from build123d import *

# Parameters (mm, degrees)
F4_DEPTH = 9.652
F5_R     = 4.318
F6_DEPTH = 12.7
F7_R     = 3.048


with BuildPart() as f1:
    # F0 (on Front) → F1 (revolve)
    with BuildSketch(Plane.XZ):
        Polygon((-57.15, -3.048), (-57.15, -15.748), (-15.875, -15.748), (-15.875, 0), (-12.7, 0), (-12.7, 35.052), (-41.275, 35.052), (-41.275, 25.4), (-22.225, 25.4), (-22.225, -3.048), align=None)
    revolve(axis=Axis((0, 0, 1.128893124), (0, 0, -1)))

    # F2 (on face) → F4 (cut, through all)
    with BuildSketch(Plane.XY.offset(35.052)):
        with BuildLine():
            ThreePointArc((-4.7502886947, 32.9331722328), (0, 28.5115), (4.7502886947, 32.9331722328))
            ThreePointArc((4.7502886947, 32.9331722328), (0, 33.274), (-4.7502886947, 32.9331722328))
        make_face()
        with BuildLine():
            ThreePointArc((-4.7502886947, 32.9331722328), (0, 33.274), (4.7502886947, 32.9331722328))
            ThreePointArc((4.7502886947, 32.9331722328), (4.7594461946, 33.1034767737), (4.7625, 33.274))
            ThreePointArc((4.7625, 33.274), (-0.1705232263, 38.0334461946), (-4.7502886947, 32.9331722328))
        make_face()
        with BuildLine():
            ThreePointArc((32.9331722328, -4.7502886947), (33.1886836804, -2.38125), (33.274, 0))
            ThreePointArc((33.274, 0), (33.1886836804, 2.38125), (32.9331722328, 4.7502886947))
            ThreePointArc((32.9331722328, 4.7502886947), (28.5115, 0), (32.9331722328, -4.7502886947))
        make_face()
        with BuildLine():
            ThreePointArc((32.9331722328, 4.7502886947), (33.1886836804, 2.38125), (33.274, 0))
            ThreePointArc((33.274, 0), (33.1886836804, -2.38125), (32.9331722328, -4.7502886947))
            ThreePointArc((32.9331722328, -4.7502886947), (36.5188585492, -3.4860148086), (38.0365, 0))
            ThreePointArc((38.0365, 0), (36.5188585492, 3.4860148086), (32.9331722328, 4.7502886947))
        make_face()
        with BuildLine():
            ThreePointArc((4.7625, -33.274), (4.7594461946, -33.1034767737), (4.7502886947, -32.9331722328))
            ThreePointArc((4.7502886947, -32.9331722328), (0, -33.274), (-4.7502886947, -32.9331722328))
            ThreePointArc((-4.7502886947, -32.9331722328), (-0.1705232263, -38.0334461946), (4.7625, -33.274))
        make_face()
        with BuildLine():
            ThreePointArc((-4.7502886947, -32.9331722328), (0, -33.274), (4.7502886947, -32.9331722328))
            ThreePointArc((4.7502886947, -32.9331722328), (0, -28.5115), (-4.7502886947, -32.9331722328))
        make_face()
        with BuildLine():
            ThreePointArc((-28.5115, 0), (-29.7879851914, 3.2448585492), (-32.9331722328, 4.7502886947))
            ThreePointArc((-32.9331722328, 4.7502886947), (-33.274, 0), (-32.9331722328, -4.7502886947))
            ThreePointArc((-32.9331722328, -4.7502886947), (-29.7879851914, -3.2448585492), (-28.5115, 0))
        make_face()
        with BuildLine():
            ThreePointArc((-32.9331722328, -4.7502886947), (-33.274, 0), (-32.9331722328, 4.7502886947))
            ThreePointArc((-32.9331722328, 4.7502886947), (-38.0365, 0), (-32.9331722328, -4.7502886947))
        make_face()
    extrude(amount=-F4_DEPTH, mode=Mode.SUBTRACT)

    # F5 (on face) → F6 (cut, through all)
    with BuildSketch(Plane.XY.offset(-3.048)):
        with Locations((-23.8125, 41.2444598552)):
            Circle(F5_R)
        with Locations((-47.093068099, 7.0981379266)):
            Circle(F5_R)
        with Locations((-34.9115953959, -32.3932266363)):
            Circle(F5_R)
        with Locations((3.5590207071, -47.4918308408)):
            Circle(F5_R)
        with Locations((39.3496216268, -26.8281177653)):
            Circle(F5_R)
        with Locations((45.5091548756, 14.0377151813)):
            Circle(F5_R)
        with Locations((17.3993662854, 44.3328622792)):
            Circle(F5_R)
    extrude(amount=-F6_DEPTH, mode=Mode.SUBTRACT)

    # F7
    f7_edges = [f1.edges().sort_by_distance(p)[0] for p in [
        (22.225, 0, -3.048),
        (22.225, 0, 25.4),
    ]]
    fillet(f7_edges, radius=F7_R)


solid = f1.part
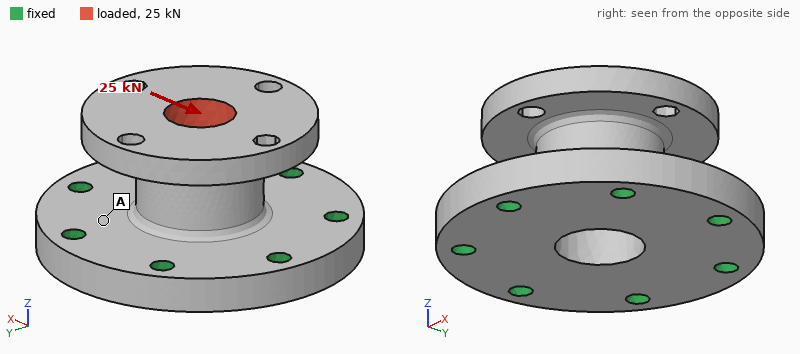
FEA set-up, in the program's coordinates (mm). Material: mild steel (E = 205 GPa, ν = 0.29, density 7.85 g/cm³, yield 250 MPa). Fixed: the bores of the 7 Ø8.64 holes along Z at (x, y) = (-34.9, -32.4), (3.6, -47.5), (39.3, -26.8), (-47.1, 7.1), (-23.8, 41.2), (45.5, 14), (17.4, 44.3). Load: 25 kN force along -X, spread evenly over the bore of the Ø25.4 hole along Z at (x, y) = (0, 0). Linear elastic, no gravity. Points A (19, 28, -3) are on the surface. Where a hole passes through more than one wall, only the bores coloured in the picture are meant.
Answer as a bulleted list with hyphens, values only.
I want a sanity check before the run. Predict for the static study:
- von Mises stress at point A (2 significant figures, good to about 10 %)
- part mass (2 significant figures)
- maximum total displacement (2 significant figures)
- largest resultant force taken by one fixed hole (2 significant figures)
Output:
- 24 MPa
- 1.5 kg
- 51 µm
- 7.7 kN
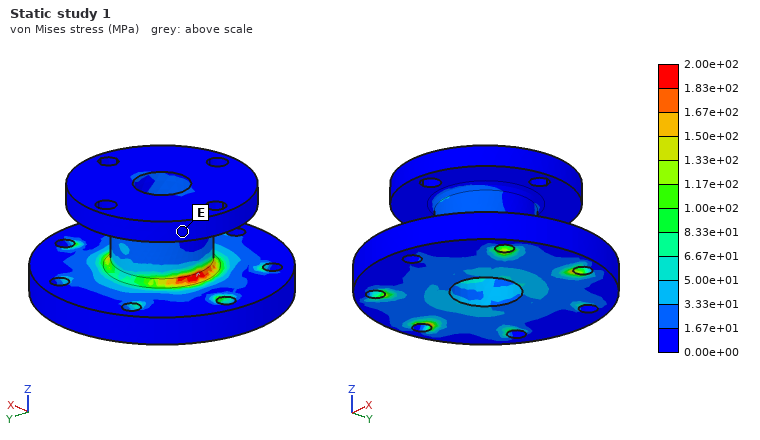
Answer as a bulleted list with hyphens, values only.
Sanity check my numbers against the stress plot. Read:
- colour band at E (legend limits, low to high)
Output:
- 0.00e+00 to 1.67e+01 MPa
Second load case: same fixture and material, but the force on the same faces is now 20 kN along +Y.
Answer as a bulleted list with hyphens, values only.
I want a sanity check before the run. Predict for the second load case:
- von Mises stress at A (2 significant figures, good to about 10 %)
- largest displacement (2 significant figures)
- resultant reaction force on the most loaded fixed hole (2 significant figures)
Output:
- 24 MPa
- 41 µm
- 6.2 kN
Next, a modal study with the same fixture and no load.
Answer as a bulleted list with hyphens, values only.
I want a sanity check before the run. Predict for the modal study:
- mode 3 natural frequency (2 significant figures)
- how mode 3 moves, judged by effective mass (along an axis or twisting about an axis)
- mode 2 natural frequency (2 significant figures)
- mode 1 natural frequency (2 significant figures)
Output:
- 6900 Hz
- along Z
- 4400 Hz
- 4400 Hz
